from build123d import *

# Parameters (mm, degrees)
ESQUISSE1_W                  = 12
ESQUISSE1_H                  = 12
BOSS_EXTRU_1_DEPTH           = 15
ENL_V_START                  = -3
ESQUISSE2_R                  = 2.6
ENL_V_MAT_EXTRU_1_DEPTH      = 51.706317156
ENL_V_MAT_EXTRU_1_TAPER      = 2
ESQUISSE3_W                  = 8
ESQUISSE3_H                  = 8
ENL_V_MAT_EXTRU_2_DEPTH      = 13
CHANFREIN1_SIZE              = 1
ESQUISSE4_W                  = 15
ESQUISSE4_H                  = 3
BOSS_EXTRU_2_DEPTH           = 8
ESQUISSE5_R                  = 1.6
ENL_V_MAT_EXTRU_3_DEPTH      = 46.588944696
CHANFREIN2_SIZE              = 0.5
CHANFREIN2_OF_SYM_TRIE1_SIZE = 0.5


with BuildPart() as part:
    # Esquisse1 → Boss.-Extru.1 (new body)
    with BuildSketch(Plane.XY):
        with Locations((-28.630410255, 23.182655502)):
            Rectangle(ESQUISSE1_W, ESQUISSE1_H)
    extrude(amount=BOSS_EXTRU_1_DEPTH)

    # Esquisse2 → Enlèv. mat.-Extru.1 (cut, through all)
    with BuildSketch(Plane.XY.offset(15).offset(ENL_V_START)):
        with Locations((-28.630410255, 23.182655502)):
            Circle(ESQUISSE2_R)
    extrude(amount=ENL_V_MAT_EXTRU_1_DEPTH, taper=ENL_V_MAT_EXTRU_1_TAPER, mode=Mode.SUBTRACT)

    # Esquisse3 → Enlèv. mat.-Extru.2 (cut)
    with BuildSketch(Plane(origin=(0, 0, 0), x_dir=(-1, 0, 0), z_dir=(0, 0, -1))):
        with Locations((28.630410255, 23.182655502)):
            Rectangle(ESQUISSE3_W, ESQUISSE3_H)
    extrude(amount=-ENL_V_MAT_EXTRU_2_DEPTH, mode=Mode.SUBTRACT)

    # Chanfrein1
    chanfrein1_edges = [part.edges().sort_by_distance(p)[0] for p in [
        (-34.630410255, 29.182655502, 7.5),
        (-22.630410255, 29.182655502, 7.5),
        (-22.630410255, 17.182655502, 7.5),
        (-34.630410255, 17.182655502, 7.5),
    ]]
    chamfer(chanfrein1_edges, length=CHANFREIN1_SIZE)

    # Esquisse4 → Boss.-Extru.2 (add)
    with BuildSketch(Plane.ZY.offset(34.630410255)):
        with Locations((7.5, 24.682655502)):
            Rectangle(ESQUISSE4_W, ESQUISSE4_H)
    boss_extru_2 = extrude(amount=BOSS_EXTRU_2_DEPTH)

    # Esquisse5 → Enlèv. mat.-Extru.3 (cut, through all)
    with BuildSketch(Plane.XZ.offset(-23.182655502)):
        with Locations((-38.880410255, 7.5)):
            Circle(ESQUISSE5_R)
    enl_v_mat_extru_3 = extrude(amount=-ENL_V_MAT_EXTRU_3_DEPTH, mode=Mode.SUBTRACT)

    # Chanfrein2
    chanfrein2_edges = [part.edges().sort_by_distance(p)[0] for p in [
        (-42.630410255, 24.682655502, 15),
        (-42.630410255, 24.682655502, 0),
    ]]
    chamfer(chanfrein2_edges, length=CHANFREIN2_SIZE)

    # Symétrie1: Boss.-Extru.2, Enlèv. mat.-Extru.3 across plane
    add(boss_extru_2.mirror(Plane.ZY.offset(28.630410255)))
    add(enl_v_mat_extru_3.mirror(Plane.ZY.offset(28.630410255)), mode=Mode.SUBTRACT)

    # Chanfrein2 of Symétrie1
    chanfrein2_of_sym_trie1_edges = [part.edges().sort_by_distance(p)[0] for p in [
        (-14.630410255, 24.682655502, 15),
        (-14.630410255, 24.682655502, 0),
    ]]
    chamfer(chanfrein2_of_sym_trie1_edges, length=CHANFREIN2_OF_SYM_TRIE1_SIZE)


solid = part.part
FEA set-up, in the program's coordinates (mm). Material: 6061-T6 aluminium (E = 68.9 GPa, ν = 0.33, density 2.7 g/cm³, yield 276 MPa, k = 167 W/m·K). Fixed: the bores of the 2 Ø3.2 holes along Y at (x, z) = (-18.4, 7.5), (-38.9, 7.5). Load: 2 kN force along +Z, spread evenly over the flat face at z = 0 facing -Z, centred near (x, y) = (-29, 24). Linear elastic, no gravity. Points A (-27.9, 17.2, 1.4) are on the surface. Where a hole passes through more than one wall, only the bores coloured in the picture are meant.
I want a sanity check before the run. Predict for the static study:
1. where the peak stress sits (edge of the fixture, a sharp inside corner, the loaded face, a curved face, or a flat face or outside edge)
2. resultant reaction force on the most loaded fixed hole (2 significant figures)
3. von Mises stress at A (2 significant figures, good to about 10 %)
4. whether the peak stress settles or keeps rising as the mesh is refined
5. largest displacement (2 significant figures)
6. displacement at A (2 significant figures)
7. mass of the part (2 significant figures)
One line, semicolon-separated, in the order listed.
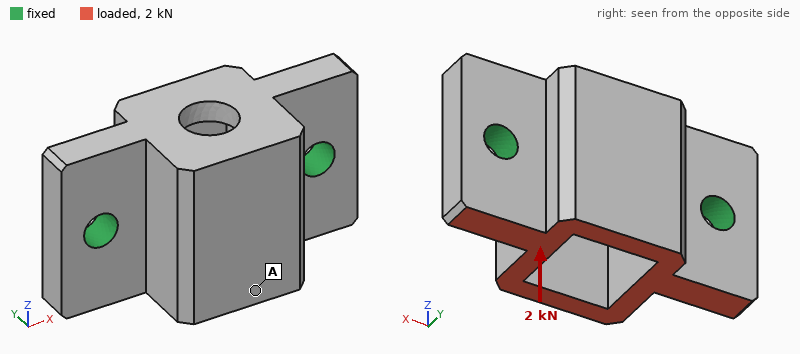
edge of the fixture; 1.0 kN; 16 MPa; keeps rising; 20 µm; 19 µm; 5.2 g
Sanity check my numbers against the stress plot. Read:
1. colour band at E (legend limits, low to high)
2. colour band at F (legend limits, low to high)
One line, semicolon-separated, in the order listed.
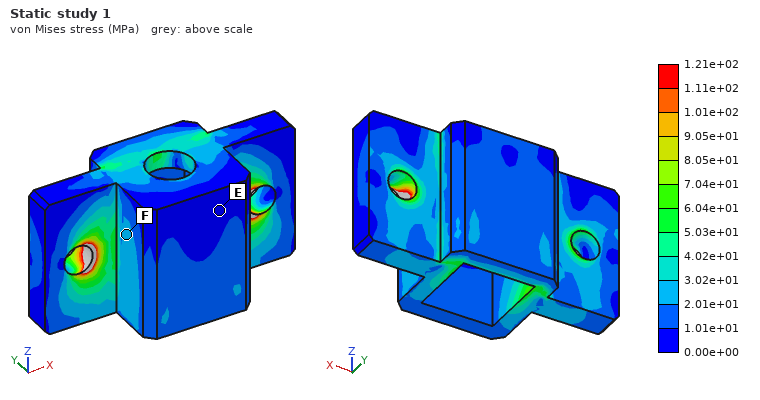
0.00e+00 to 1.01e+01 MPa; 2.01e+01 to 3.02e+01 MPa
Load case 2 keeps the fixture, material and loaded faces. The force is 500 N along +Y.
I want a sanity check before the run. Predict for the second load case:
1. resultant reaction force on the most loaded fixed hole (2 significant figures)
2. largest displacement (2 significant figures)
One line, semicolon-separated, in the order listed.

250 N; 25 µm
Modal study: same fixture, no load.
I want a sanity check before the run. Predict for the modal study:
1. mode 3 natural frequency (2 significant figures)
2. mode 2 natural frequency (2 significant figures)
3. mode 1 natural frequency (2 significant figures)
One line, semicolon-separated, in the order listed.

32 kHz; 31 kHz; 17 kHz
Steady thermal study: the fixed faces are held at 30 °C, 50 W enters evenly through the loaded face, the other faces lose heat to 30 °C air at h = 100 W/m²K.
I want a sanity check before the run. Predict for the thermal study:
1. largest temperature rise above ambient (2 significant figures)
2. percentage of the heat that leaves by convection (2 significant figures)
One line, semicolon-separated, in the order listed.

34 K; 5.2 %
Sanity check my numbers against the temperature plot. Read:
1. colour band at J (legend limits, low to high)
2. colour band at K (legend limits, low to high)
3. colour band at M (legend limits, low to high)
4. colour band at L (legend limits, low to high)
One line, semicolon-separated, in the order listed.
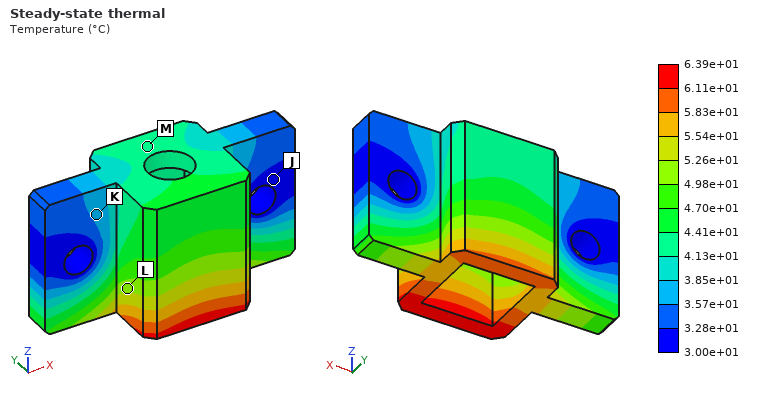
3.00e+01 to 3.28e+01 °C; 3.57e+01 to 3.85e+01 °C; 4.13e+01 to 4.41e+01 °C; 4.98e+01 to 5.26e+01 °C
